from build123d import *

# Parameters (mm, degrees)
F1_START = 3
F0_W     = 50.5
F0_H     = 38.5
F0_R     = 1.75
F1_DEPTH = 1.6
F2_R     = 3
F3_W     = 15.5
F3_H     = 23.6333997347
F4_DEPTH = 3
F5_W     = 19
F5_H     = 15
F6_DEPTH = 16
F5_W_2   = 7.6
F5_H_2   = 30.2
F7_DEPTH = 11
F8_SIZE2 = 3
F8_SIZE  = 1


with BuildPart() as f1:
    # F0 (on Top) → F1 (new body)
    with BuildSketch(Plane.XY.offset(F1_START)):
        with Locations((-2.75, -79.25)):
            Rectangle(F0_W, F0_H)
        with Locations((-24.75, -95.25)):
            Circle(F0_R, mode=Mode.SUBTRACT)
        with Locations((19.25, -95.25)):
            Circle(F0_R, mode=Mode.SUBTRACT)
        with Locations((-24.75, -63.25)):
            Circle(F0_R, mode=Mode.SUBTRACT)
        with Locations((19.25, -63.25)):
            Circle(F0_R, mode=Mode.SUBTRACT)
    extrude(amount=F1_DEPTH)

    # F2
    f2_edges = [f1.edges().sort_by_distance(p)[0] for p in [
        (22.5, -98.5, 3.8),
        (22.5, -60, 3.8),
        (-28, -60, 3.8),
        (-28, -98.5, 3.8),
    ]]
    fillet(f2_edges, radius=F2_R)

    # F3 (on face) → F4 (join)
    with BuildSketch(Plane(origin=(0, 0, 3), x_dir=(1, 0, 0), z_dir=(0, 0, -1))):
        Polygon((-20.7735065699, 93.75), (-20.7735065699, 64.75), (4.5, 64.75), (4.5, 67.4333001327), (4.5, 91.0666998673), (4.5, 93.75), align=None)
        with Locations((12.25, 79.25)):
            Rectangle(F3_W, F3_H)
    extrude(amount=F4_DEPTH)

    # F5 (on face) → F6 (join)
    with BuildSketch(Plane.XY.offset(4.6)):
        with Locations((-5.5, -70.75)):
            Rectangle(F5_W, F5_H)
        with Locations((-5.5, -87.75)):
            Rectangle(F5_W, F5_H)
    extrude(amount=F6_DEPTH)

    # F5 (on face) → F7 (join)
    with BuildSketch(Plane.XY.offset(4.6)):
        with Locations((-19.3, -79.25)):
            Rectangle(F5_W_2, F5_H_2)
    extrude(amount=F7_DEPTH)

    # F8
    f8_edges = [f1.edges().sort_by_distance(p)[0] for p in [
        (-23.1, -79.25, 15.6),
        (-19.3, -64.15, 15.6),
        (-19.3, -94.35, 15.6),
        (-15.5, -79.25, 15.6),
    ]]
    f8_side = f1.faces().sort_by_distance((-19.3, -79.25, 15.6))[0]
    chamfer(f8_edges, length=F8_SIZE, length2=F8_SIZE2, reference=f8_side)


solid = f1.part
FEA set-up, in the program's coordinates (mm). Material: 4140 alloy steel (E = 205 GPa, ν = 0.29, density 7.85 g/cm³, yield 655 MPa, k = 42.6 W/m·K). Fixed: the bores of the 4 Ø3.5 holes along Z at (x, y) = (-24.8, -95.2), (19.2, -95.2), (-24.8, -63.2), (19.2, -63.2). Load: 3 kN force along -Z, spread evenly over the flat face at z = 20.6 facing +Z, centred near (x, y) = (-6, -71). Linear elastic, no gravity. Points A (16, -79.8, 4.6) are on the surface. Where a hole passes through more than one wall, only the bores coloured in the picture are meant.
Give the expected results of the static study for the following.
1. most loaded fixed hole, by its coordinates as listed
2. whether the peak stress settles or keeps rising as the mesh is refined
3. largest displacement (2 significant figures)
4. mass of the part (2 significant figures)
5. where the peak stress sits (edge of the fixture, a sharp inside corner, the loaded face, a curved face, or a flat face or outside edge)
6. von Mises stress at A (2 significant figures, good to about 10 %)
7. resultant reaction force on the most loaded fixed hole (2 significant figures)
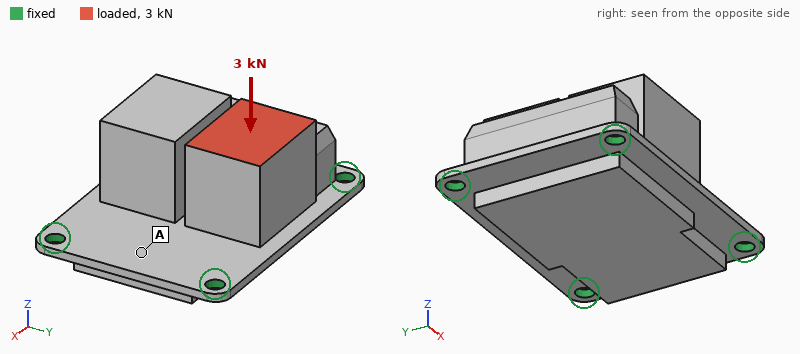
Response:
(-24.8, -63.2)
keeps rising
57 µm
140 g
edge of the fixture
41 MPa
1.5 kN
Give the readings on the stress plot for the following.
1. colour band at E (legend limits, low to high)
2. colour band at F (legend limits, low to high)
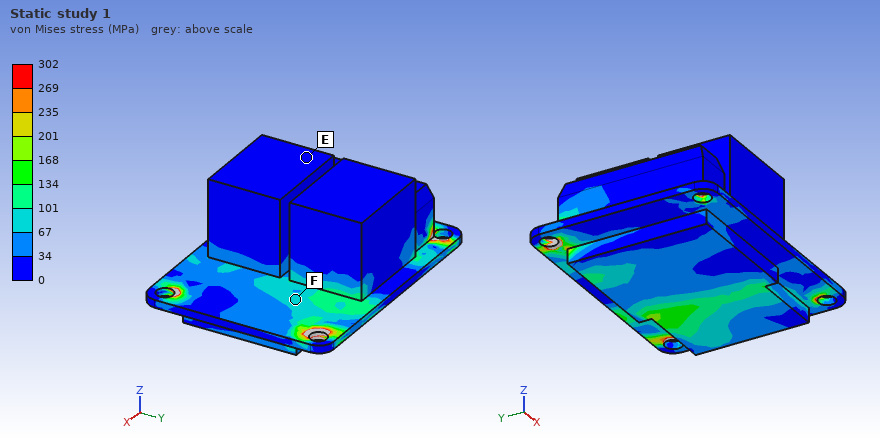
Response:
0 to 34 MPa
67 to 101 MPa
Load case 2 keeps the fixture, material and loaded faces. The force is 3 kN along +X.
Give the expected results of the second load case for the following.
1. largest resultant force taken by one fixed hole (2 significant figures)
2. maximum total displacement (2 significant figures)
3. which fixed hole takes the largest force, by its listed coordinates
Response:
1.7 kN
56 µm
(-24.8, -63.2)
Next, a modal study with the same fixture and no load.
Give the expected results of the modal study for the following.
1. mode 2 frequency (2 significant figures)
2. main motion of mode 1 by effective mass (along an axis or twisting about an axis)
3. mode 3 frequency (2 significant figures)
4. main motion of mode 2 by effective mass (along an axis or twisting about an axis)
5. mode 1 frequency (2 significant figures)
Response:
6400 Hz
along Z
8700 Hz
along Y
4400 Hz
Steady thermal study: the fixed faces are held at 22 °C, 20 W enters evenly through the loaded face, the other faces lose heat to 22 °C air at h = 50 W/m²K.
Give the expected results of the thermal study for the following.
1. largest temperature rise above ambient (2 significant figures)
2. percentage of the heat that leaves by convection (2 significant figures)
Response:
61 K
44 %
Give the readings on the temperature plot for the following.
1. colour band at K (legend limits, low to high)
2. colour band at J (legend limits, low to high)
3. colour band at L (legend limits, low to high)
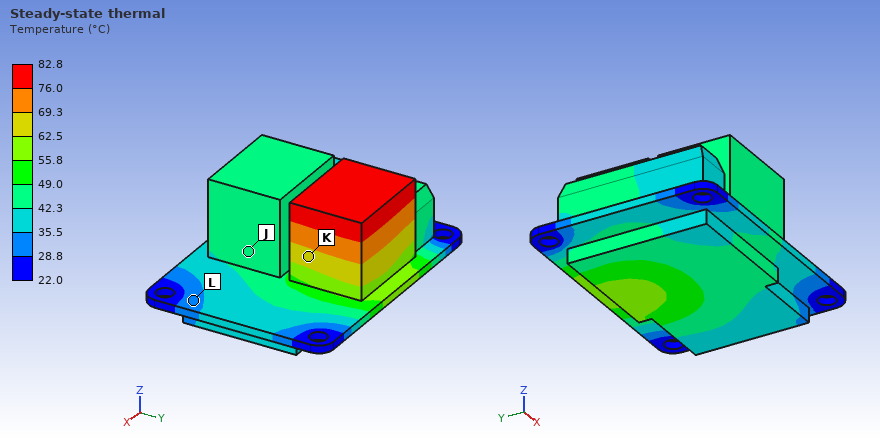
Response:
62.5 to 69.3 °C
42.3 to 49.0 °C
28.8 to 35.5 °C
